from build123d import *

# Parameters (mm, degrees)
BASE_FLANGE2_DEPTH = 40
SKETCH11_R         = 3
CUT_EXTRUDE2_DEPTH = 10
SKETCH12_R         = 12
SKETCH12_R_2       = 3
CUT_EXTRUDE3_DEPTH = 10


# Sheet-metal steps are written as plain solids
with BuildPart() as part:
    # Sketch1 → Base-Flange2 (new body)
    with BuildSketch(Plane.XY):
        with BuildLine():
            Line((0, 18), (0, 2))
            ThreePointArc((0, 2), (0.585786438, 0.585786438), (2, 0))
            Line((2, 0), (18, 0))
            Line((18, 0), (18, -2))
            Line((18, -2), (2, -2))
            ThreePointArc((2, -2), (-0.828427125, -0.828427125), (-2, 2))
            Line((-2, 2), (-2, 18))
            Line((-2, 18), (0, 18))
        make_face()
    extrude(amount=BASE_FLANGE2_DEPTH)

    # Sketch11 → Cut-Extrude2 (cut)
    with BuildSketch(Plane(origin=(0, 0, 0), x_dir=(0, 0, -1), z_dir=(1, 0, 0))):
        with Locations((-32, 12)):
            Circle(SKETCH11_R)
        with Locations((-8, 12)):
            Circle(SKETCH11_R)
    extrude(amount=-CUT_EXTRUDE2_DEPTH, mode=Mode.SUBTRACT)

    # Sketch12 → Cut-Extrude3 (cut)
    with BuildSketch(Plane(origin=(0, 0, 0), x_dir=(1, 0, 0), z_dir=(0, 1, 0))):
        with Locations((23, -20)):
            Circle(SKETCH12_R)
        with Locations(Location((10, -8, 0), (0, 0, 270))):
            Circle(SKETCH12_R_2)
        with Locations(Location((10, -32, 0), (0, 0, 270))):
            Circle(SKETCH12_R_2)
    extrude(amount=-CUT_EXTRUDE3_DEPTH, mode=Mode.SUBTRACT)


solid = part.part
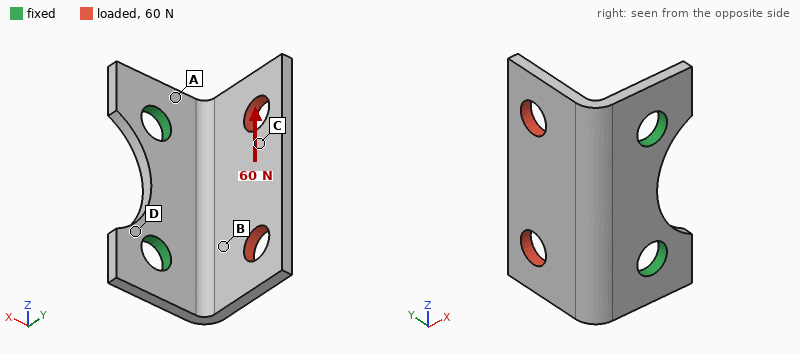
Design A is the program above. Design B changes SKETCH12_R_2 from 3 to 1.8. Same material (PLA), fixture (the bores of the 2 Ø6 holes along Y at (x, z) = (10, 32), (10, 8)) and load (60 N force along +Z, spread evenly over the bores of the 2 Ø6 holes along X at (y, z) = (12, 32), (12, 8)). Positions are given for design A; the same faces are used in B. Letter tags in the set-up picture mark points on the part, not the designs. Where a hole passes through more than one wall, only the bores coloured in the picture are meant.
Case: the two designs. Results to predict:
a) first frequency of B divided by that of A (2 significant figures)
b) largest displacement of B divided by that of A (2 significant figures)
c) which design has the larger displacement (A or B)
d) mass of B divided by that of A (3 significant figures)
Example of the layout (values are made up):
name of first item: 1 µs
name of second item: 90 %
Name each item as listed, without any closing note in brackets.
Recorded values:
first frequency of B divided by that of A: 0.91
largest displacement of B divided by that of A: 1.3
which design has the larger displacement: B
mass of B divided by that of A: 1.03
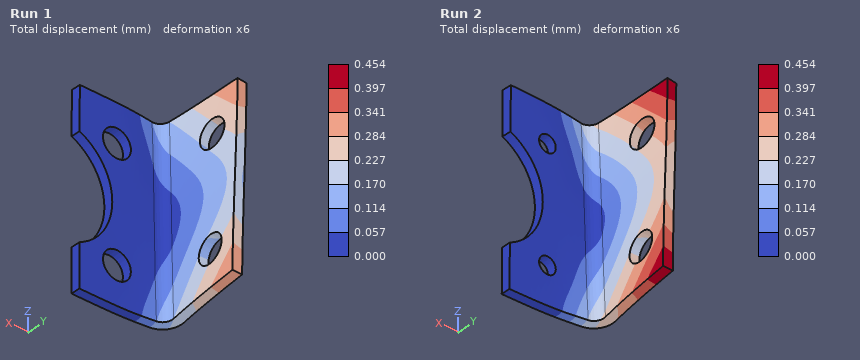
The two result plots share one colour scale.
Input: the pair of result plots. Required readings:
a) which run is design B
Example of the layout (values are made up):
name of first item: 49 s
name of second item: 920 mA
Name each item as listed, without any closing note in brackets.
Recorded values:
which run is design B: Run 2
